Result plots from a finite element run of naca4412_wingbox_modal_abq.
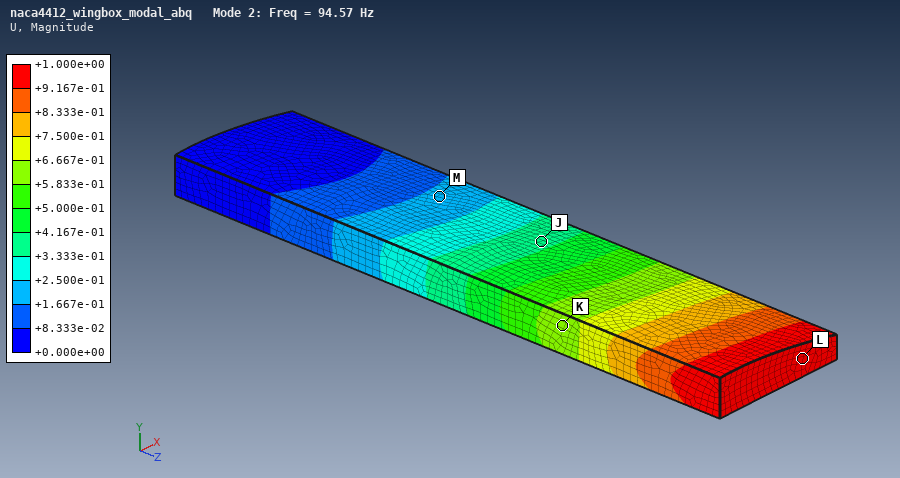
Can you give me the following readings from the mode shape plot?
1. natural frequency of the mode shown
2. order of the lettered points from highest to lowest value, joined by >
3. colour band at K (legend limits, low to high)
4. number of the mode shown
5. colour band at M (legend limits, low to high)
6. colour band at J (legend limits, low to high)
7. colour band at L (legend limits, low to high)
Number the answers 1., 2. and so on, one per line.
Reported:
1. 94.57 Hz
2. L > K > J > M
3. +5.833e-01 to +6.667e-01
4. 2
5. +1.667e-01 to +2.500e-01
6. +3.333e-01 to +4.167e-01
7. +9.167e-01 to +1.000e+00
